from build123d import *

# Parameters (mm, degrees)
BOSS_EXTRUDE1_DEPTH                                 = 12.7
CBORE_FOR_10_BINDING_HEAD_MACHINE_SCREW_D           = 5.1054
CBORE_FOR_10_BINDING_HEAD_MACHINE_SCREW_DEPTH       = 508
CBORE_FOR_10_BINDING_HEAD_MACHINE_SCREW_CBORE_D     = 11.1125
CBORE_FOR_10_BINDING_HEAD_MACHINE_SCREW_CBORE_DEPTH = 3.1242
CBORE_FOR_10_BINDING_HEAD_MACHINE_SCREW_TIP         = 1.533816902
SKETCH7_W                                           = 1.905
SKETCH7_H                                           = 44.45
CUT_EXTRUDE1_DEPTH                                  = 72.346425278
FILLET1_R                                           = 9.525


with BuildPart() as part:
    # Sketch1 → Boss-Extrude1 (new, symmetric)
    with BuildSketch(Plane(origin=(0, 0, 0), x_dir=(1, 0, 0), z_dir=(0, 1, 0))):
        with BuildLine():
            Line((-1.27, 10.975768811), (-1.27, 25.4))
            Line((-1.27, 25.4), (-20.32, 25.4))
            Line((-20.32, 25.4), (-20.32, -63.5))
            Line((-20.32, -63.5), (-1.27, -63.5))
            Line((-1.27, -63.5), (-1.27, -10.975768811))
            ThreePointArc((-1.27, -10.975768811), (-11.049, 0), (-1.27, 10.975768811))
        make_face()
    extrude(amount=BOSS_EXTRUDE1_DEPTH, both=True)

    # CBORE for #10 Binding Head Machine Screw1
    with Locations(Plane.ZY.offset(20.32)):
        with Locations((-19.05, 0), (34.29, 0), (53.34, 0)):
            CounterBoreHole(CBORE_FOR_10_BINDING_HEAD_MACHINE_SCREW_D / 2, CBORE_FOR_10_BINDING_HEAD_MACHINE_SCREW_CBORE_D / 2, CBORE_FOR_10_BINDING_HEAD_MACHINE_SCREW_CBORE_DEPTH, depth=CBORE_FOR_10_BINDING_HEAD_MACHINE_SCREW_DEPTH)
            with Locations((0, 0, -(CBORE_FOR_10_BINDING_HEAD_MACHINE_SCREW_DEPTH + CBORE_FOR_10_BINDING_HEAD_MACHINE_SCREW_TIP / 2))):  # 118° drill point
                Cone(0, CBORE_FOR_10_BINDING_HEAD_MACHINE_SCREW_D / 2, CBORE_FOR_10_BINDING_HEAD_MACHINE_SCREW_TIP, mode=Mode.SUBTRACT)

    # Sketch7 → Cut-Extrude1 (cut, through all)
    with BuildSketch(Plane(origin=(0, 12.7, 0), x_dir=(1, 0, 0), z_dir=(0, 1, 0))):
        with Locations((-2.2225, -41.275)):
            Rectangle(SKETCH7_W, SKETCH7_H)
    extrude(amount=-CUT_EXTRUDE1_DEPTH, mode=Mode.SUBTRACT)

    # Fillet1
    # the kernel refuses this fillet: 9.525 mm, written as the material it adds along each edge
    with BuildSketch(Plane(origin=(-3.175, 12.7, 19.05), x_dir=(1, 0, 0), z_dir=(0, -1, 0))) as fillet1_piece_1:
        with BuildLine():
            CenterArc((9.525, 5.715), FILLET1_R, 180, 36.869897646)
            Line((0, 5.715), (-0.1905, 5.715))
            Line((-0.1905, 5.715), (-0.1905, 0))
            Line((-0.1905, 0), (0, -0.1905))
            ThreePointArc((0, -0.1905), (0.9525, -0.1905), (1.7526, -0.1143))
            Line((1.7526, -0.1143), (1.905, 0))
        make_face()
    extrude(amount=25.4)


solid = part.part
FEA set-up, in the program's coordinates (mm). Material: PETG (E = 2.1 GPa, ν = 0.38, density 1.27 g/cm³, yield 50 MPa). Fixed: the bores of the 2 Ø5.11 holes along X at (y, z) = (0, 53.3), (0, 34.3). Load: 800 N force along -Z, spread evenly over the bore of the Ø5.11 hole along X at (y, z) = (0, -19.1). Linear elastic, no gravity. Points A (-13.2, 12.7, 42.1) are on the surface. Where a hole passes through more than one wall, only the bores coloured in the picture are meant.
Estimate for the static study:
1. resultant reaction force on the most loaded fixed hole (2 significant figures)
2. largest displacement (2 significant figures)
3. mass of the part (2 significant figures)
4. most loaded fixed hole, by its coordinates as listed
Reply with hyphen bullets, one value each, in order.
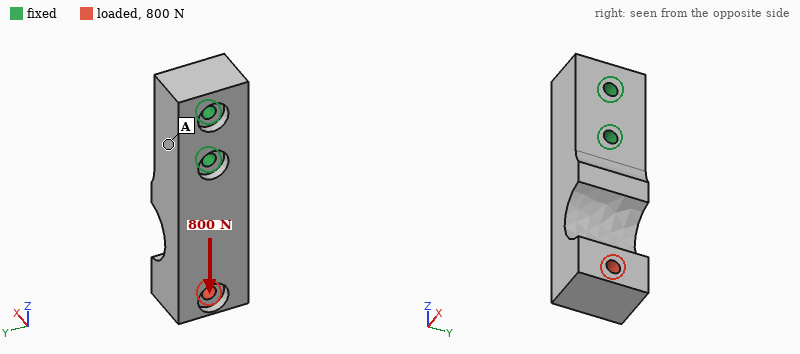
- 640 N
- 0.77 mm
- 44 g
- (0, 34.3)
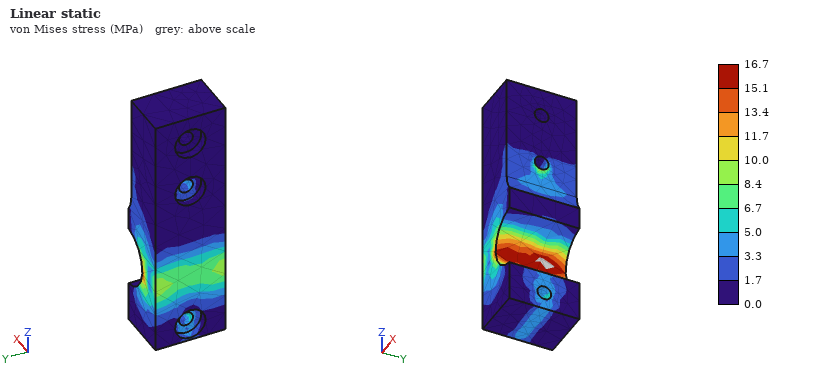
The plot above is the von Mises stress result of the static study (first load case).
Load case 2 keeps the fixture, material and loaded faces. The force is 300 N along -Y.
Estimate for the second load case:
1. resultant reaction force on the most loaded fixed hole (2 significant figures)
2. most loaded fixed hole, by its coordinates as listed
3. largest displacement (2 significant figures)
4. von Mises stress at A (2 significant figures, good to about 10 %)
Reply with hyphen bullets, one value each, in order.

- 890 N
- (0, 34.3)
- 0.88 mm
- 4.6 MPa
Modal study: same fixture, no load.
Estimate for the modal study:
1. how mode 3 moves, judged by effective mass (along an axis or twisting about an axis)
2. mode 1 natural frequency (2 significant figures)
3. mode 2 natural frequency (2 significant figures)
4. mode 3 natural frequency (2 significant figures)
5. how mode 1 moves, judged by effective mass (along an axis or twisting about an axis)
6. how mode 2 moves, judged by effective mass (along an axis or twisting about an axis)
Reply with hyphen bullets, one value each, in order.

- twisting about Z
- 750 Hz
- 1000 Hz
- 2200 Hz
- along X
- along Y
